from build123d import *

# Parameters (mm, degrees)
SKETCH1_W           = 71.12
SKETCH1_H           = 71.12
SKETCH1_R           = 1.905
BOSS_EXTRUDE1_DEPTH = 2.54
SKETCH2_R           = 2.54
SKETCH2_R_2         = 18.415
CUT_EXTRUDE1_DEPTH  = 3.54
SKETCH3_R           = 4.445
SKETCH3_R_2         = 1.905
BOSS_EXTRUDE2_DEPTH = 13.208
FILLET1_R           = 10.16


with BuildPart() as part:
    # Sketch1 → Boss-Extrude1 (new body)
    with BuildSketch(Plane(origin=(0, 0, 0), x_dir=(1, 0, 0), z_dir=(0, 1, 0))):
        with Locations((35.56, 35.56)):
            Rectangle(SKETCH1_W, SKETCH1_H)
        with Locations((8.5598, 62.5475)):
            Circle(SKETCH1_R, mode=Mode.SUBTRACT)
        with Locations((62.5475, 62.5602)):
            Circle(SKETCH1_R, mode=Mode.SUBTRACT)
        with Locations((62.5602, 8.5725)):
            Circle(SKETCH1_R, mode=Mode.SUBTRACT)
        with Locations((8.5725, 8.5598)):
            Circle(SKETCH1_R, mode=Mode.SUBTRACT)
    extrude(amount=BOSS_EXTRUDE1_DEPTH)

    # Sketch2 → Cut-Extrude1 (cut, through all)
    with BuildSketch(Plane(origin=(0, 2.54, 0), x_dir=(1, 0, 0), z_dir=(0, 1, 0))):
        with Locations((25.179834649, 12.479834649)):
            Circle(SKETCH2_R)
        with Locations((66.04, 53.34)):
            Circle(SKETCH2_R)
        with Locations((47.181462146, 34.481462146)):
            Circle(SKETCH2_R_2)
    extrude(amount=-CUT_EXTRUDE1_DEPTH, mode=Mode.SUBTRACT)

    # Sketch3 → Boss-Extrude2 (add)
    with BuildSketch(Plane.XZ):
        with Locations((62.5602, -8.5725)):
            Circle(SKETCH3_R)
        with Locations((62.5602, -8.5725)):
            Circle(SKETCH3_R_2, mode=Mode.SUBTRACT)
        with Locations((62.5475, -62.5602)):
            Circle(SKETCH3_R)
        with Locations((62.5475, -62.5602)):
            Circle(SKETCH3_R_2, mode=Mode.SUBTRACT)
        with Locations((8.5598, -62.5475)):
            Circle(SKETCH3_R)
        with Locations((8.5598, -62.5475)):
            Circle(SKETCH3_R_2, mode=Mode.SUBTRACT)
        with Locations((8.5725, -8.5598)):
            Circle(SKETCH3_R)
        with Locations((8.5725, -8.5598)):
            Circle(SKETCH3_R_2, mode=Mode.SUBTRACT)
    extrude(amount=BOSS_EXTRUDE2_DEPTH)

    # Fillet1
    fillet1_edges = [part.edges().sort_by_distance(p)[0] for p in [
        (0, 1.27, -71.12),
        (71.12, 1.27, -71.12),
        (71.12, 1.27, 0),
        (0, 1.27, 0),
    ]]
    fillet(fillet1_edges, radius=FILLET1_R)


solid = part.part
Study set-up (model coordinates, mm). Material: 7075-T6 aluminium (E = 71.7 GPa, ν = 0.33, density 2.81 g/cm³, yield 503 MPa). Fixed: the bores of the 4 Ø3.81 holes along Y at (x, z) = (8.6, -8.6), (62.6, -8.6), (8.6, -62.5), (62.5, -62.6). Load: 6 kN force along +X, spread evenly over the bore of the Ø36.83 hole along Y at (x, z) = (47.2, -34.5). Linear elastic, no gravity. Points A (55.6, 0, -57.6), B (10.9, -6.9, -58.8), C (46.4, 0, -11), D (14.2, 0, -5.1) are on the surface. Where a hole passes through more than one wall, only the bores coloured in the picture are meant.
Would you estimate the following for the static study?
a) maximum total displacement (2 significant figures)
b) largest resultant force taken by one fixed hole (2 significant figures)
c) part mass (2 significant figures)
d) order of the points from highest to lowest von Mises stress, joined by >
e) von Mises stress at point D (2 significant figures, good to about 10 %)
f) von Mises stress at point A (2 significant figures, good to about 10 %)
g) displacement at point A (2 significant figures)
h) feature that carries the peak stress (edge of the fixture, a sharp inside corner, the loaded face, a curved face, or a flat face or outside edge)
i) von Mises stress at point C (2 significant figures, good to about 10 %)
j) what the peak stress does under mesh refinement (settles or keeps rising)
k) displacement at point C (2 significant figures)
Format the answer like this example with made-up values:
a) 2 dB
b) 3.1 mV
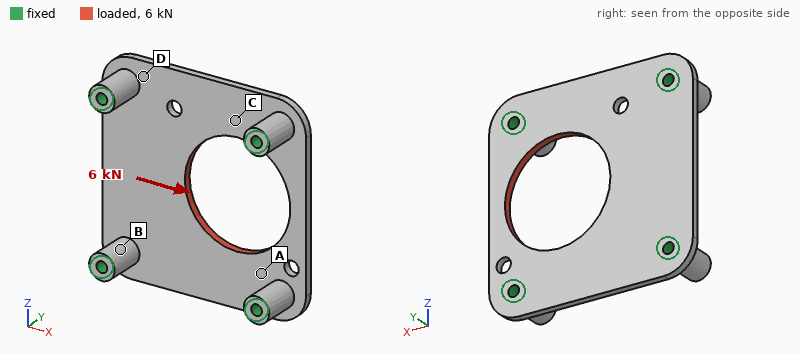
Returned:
a) 62 µm
b) 1.9 kN
c) 35 g
d) A > C > D > B
e) 23 MPa
f) 56 MPa
g) 11 µm
h) edge of the fixture
i) 36 MPa
j) keeps rising
k) 11 µm
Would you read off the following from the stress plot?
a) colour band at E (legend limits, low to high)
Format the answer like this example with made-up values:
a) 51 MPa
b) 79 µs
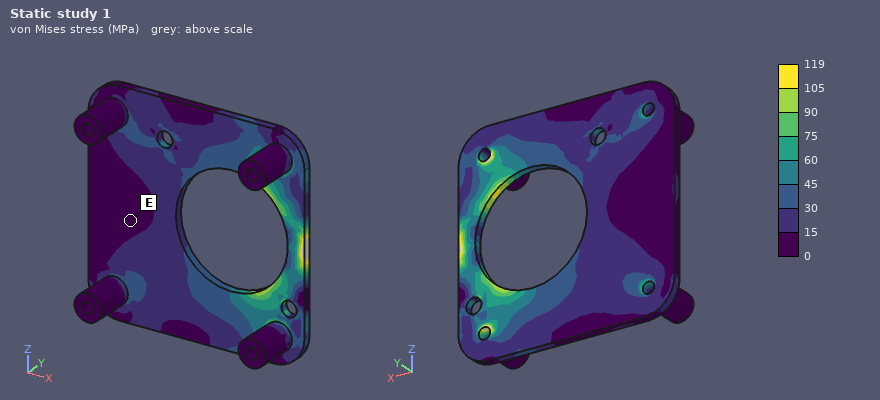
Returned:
a) 0 to 15 MPa
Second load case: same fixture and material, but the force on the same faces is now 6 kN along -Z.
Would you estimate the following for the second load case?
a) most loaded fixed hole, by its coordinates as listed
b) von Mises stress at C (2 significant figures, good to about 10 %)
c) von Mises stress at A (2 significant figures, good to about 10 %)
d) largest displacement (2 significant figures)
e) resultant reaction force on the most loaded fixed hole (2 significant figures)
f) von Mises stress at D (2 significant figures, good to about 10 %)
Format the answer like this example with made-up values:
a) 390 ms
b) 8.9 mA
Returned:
a) (62.6, -8.6)
b) 22 MPa
c) 32 MPa
d) 23 µm
e) 1.9 kN
f) 18 MPa
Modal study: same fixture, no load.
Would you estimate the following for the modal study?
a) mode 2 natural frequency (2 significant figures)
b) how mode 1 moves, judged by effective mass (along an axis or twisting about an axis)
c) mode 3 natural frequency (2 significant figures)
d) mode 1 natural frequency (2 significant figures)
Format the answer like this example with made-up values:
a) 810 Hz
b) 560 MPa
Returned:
a) 5500 Hz
b) along Y
c) 5600 Hz
d) 4000 Hz
